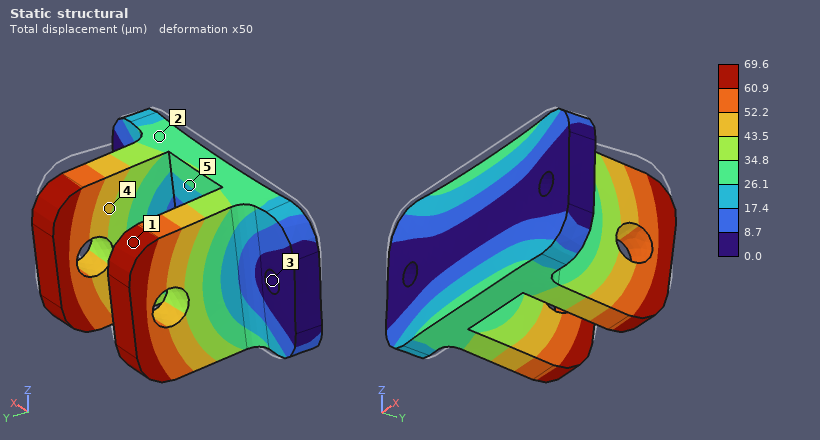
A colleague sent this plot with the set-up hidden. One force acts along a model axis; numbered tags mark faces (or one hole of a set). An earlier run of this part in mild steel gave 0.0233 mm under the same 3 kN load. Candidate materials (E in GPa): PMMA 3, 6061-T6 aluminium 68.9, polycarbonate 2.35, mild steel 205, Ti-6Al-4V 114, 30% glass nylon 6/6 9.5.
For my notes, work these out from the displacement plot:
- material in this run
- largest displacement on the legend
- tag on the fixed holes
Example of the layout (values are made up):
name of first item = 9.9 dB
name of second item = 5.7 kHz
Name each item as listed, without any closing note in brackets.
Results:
material in this run = 6061-T6 aluminium
largest displacement on the legend = 69.6 µm
tag on the fixed holes = 3
